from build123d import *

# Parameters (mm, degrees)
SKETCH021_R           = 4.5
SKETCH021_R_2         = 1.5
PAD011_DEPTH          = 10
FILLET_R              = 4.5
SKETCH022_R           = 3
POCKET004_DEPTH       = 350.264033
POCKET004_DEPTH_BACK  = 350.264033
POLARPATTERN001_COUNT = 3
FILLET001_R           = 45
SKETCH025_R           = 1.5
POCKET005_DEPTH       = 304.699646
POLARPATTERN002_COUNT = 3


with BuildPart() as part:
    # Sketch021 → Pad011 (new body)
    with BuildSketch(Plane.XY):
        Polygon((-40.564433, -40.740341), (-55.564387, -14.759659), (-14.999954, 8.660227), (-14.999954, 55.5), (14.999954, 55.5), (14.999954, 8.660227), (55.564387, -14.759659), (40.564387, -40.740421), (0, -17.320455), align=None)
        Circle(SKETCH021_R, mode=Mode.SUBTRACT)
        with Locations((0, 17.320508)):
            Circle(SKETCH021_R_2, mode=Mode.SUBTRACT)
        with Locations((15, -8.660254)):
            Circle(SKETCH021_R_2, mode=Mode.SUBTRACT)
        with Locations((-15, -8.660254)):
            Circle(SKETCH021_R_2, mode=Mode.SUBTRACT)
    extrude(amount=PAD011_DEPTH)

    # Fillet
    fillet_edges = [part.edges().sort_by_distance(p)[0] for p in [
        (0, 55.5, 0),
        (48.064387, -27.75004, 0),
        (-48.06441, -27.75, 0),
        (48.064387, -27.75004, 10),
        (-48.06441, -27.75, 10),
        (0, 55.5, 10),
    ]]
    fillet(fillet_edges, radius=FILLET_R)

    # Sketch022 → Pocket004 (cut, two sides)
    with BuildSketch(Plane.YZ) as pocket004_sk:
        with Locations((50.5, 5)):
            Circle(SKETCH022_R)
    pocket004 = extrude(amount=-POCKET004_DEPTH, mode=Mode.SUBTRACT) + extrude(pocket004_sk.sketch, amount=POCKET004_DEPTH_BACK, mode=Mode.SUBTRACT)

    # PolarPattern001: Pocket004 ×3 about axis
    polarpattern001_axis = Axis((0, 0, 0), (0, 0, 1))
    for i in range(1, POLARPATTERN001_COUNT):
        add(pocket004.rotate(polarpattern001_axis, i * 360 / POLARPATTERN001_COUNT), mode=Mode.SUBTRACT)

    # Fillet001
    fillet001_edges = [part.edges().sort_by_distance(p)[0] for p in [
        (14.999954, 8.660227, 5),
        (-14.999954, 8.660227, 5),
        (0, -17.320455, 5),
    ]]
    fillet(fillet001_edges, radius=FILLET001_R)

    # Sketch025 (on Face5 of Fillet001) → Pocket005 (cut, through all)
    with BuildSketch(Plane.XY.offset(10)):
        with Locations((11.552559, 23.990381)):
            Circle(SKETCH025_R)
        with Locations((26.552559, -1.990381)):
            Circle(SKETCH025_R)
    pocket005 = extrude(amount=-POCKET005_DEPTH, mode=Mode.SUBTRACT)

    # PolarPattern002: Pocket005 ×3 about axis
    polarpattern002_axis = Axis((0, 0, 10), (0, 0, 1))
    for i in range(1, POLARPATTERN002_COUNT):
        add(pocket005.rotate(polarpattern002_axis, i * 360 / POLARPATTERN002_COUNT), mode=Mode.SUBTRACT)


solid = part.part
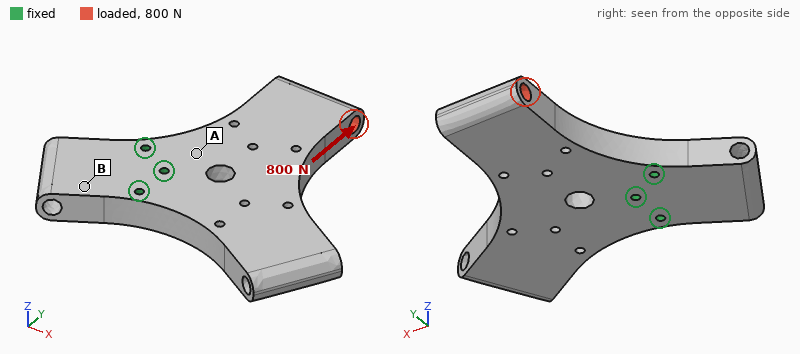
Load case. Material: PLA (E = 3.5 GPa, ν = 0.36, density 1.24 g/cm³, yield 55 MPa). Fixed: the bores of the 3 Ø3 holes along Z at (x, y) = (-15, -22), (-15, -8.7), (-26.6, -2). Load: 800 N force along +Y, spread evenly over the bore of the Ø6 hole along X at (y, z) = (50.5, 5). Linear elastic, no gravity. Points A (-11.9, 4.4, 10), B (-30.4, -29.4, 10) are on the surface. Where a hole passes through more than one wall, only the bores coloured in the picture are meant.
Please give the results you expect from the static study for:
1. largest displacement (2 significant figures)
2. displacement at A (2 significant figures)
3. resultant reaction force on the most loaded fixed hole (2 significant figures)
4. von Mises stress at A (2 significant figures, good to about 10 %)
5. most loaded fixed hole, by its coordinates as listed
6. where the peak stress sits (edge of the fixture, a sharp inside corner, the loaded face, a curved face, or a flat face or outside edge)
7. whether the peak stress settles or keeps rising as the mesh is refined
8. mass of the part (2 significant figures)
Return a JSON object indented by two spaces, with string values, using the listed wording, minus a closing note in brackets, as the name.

{
  "largest displacement": "0.22 mm",
  "displacement at A": "0.035 mm",
  "resultant reaction force on the most loaded fixed hole": "690 N",
  "von Mises stress at A": "4.3 MPa",
  "most loaded fixed hole, by its coordinates as listed": "(-15, -8.7)",
  "where the peak stress sits": "edge of the fixture",
  "whether the peak stress settles or keeps rising as the mesh is refined": "keeps rising",
  "mass of the part": "55 g"
}
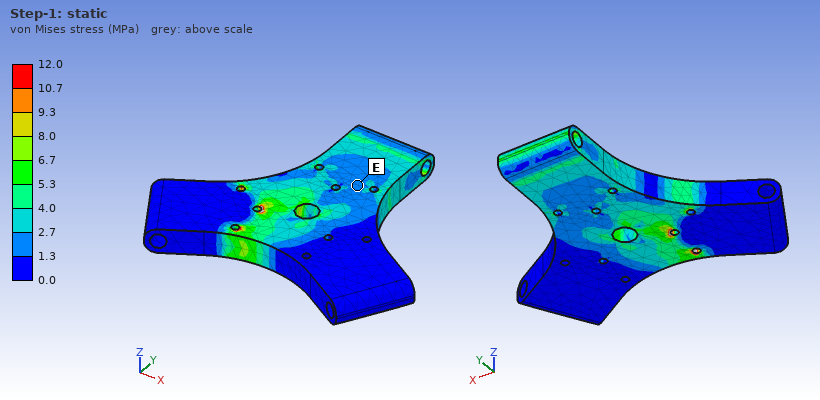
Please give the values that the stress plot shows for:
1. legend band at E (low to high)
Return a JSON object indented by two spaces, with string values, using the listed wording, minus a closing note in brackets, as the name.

{
  "legend band at E": "1.3 to 2.7 MPa"
}
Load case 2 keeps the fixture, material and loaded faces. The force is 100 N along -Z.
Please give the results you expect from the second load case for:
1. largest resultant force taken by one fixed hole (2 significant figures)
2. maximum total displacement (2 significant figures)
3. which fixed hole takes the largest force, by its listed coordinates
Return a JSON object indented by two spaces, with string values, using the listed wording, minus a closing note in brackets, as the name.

{
  "largest resultant force taken by one fixed hole": "180 N",
  "maximum total displacement": "0.96 mm",
  "which fixed hole takes the largest force, by its listed coordinates": "(-15, -8.7)"
}
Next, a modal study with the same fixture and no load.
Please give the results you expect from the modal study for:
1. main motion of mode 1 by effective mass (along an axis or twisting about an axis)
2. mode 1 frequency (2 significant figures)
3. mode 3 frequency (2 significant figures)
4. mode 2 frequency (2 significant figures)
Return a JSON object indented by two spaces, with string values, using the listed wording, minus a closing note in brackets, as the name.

{
  "main motion of mode 1 by effective mass": "along Z",
  "mode 1 frequency": "640 Hz",
  "mode 3 frequency": "1300 Hz",
  "mode 2 frequency": "710 Hz"
}
